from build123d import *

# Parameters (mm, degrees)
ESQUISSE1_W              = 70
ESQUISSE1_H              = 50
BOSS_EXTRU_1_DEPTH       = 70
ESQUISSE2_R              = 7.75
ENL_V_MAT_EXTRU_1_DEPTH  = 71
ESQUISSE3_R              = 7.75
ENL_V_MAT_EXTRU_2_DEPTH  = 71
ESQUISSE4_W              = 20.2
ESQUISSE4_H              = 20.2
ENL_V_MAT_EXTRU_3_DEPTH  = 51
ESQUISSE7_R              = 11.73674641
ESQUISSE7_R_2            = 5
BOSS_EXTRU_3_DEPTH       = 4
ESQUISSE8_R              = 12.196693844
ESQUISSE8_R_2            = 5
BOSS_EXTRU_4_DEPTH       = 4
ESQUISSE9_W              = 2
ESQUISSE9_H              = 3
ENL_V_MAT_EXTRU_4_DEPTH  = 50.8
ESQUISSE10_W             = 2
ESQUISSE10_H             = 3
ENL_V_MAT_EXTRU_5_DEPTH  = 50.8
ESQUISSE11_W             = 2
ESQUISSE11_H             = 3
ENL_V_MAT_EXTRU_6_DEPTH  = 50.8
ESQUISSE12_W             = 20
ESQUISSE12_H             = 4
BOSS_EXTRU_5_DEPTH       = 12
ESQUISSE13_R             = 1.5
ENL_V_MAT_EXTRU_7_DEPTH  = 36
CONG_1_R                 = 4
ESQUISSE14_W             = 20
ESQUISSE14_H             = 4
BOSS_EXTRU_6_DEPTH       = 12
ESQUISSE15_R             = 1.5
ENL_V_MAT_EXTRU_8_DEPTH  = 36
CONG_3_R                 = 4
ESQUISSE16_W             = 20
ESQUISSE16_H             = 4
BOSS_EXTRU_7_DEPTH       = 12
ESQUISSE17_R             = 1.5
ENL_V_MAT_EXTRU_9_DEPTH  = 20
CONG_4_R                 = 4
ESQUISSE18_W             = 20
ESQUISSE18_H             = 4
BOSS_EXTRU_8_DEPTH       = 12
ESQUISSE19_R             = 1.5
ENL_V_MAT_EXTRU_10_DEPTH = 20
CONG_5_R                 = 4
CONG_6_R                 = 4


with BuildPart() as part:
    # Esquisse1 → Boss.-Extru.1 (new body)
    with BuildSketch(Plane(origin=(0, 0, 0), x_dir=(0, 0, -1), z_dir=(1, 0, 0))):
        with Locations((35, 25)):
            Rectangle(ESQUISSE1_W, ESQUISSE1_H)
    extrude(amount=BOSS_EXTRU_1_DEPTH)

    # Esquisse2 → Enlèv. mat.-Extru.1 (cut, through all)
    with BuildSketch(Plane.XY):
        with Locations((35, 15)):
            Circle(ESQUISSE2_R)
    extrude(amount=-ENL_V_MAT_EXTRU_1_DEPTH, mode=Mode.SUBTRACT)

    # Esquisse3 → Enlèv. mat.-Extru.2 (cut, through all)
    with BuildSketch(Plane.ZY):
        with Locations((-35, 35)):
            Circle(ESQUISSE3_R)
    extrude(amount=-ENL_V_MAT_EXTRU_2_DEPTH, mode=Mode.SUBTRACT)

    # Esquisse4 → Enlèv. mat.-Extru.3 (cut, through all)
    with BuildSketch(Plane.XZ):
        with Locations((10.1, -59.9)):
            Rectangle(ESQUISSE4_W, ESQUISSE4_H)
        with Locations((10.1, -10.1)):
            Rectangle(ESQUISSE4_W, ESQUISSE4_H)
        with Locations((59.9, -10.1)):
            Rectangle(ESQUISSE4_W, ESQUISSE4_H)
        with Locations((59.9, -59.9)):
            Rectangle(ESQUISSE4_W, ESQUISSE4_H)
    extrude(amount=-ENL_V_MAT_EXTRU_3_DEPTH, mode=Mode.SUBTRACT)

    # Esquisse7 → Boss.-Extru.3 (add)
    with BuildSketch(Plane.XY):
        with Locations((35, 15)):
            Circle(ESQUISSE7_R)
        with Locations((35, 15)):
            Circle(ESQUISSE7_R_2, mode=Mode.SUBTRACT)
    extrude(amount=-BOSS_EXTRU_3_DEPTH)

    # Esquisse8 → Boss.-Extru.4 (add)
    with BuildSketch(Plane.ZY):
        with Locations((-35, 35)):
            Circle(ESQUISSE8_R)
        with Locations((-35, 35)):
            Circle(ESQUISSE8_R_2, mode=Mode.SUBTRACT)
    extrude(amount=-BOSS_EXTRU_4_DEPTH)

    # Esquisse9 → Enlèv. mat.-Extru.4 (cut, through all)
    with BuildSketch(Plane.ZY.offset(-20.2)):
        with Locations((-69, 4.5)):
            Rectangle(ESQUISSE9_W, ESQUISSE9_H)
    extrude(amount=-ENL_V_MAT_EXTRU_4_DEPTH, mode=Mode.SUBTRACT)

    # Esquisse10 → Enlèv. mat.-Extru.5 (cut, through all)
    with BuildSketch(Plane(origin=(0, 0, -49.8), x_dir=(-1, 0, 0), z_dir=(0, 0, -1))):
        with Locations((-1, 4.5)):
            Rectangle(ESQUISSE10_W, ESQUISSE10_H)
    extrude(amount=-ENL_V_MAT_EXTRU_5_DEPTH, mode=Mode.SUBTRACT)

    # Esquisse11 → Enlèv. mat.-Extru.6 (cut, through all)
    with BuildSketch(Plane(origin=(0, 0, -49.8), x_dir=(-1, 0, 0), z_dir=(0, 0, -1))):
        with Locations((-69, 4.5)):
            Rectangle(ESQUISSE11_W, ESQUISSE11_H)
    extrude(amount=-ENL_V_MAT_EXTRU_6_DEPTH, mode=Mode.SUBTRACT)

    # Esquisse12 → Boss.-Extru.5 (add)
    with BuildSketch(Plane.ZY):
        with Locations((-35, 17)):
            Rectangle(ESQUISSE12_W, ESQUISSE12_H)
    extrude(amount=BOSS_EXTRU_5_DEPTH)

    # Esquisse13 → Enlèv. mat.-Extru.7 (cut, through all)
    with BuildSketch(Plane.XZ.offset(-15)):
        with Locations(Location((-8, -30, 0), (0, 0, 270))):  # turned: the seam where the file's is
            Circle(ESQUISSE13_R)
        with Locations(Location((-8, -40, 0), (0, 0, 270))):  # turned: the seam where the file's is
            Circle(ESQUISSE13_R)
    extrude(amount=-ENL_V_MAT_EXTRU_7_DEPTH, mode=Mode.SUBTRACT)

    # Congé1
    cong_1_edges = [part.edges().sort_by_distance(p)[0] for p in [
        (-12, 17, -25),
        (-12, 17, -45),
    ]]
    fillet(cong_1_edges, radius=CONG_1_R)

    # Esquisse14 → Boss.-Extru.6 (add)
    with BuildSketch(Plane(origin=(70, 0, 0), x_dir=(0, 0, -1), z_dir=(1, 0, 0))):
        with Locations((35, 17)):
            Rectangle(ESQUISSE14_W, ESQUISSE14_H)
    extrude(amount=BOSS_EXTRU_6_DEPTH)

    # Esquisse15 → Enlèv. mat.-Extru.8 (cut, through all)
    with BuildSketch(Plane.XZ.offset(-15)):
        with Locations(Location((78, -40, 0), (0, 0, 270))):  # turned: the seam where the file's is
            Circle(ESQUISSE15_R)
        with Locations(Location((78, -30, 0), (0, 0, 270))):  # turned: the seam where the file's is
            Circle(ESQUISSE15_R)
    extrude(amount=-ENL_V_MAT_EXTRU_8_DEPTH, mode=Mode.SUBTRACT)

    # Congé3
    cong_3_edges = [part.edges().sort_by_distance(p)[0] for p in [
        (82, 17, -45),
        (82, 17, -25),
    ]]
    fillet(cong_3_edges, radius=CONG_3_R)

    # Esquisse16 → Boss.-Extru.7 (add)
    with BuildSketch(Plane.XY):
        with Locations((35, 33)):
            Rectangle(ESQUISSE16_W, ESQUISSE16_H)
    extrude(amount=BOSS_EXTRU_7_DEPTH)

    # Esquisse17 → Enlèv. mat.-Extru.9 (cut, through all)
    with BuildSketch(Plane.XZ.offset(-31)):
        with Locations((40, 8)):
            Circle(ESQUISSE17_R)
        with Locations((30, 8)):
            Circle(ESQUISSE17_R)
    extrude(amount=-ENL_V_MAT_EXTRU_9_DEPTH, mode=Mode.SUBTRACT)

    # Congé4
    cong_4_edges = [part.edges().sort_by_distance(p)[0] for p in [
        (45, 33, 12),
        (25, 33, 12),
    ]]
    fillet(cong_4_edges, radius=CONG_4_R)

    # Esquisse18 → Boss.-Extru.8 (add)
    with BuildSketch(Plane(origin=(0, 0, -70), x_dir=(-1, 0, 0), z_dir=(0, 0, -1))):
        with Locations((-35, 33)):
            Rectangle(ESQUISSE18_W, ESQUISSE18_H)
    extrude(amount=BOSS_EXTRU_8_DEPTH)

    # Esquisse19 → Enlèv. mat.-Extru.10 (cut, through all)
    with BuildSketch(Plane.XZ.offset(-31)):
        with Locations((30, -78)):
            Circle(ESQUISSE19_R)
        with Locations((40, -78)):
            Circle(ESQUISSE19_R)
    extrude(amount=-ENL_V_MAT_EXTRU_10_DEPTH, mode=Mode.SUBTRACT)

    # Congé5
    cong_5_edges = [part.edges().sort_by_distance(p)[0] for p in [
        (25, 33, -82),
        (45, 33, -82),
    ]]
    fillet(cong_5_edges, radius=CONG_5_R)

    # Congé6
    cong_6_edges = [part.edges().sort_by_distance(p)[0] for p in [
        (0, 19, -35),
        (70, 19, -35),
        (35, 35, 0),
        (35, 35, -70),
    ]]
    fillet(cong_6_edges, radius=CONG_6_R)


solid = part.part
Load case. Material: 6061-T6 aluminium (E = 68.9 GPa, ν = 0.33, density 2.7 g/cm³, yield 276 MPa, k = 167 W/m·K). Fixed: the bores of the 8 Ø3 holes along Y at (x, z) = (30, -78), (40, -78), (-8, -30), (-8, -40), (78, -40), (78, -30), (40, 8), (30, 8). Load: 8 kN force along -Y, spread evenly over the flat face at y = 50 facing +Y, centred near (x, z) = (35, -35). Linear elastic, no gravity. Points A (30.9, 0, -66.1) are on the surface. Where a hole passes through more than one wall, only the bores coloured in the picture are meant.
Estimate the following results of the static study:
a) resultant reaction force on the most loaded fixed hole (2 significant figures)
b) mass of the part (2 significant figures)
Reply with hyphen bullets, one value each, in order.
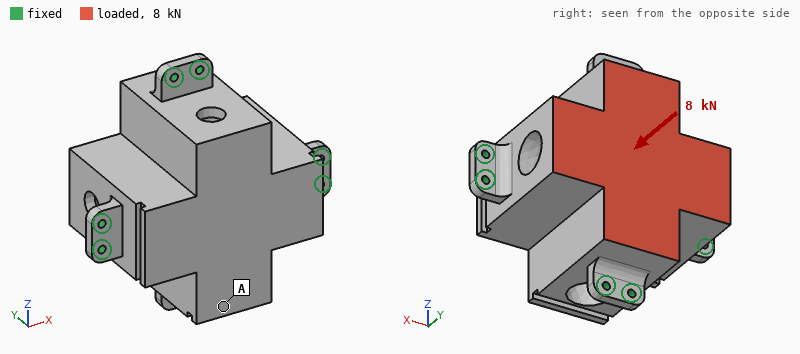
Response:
- 1.1 kN
- 380 g
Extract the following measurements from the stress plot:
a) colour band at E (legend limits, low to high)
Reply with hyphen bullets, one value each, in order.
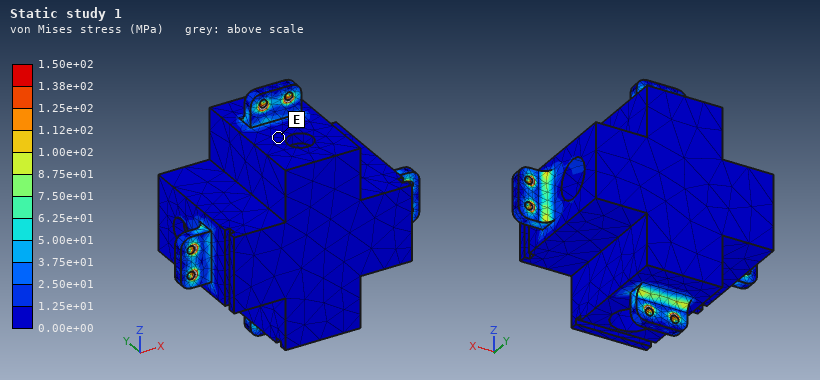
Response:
- 0.00e+00 to 1.25e+01 MPa
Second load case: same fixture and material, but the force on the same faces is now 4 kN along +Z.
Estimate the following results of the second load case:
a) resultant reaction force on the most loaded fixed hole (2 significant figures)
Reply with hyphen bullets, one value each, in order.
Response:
- 1.0 kN
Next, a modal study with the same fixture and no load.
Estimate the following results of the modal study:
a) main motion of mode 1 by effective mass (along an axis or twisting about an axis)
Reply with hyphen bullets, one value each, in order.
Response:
- along Y
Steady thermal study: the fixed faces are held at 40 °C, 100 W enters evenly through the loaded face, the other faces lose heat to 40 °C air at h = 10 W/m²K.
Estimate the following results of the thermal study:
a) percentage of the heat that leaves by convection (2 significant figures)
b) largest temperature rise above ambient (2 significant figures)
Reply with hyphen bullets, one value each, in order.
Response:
- 4.3 %
- 24 K
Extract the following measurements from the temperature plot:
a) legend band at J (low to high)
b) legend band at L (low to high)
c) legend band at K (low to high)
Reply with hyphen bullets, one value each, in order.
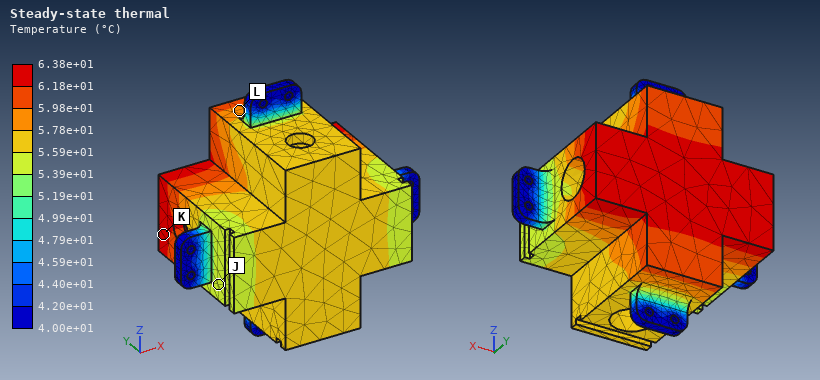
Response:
- 5.39e+01 to 5.59e+01 °C
- 5.78e+01 to 5.98e+01 °C
- 6.18e+01 to 6.38e+01 °C
